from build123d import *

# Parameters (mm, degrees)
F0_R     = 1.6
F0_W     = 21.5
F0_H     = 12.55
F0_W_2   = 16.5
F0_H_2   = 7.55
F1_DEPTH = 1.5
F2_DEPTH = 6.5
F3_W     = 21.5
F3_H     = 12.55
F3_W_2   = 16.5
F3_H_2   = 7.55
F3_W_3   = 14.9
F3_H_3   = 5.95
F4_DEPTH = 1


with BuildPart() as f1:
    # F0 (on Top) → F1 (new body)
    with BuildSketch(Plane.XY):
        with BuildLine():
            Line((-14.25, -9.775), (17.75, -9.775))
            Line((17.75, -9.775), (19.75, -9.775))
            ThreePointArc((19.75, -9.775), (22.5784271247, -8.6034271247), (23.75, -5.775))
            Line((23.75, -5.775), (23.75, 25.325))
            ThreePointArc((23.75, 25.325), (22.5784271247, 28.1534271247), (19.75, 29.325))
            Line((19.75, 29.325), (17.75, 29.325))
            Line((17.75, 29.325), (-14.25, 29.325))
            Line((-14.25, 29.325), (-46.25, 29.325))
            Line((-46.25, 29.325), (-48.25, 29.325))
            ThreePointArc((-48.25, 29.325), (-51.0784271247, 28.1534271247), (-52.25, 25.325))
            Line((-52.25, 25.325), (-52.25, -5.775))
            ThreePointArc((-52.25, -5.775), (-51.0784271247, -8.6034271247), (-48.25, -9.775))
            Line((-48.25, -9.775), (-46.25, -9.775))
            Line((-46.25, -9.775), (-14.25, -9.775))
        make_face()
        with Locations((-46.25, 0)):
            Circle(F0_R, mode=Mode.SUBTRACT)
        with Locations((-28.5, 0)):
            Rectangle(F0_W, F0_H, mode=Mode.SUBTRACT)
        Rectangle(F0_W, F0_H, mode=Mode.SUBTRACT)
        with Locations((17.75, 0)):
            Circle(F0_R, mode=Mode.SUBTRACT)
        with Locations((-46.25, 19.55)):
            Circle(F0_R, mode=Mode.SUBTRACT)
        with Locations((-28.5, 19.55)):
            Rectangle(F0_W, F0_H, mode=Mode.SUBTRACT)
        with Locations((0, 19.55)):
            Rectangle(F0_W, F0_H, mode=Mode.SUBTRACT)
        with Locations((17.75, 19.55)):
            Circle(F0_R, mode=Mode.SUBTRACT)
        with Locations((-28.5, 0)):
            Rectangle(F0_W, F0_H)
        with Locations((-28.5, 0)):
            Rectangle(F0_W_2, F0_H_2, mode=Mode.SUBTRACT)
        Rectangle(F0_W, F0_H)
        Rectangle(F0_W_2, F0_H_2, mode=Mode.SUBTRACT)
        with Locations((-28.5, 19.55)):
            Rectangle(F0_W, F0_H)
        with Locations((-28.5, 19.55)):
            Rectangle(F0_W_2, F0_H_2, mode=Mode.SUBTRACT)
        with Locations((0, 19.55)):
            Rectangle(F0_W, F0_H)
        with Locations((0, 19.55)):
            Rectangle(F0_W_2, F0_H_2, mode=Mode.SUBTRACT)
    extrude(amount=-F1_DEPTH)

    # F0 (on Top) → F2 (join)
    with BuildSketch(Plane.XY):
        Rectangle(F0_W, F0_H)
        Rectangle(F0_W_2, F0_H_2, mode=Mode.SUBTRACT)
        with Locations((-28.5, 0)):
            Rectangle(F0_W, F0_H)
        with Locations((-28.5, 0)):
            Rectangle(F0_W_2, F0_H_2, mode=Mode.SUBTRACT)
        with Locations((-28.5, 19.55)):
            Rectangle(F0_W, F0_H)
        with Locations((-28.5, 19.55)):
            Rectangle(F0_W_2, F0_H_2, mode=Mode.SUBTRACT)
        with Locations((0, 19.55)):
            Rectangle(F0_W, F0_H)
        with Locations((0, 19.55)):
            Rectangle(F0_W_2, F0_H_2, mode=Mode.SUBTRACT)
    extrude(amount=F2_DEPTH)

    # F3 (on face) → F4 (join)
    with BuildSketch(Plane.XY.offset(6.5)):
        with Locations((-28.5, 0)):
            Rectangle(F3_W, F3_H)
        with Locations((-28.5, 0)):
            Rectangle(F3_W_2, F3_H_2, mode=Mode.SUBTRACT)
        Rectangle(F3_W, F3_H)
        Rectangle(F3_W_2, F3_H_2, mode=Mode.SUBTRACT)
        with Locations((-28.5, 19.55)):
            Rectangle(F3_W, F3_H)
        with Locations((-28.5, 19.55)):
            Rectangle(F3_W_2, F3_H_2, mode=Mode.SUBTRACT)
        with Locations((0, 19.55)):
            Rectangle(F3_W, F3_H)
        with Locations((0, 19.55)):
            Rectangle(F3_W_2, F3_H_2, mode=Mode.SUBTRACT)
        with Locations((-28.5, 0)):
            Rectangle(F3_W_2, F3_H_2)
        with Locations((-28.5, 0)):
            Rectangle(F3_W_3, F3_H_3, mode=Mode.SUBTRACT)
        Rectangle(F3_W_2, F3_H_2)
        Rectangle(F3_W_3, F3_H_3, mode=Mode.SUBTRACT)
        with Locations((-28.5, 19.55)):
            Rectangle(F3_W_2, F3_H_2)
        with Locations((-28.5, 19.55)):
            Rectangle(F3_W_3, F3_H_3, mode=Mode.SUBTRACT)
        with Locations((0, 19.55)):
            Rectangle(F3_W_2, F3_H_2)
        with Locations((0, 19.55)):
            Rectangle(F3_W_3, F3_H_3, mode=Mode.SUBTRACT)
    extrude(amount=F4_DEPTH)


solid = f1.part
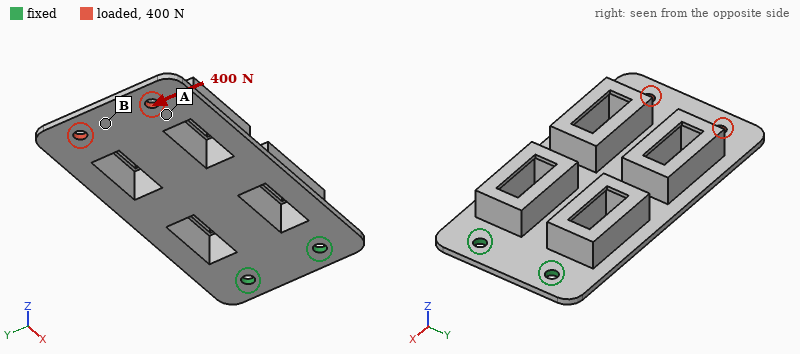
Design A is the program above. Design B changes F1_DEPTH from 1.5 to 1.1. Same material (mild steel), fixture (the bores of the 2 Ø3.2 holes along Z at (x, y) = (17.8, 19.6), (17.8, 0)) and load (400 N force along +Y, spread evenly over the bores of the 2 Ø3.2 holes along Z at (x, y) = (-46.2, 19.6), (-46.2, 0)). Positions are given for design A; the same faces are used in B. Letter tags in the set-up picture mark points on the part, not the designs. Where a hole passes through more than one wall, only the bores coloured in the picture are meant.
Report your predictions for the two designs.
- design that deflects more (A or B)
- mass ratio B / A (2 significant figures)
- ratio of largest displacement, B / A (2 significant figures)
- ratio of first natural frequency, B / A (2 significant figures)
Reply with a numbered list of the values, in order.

1. B
2. 0.88
3. 1.3
4. 0.70
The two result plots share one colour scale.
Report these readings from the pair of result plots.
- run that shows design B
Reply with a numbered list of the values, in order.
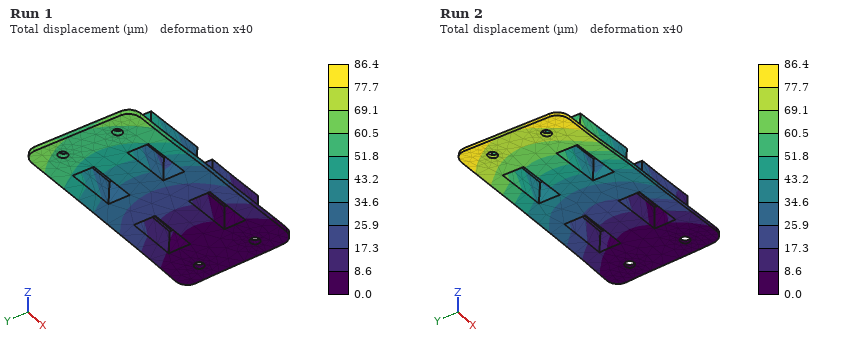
1. Run 2
